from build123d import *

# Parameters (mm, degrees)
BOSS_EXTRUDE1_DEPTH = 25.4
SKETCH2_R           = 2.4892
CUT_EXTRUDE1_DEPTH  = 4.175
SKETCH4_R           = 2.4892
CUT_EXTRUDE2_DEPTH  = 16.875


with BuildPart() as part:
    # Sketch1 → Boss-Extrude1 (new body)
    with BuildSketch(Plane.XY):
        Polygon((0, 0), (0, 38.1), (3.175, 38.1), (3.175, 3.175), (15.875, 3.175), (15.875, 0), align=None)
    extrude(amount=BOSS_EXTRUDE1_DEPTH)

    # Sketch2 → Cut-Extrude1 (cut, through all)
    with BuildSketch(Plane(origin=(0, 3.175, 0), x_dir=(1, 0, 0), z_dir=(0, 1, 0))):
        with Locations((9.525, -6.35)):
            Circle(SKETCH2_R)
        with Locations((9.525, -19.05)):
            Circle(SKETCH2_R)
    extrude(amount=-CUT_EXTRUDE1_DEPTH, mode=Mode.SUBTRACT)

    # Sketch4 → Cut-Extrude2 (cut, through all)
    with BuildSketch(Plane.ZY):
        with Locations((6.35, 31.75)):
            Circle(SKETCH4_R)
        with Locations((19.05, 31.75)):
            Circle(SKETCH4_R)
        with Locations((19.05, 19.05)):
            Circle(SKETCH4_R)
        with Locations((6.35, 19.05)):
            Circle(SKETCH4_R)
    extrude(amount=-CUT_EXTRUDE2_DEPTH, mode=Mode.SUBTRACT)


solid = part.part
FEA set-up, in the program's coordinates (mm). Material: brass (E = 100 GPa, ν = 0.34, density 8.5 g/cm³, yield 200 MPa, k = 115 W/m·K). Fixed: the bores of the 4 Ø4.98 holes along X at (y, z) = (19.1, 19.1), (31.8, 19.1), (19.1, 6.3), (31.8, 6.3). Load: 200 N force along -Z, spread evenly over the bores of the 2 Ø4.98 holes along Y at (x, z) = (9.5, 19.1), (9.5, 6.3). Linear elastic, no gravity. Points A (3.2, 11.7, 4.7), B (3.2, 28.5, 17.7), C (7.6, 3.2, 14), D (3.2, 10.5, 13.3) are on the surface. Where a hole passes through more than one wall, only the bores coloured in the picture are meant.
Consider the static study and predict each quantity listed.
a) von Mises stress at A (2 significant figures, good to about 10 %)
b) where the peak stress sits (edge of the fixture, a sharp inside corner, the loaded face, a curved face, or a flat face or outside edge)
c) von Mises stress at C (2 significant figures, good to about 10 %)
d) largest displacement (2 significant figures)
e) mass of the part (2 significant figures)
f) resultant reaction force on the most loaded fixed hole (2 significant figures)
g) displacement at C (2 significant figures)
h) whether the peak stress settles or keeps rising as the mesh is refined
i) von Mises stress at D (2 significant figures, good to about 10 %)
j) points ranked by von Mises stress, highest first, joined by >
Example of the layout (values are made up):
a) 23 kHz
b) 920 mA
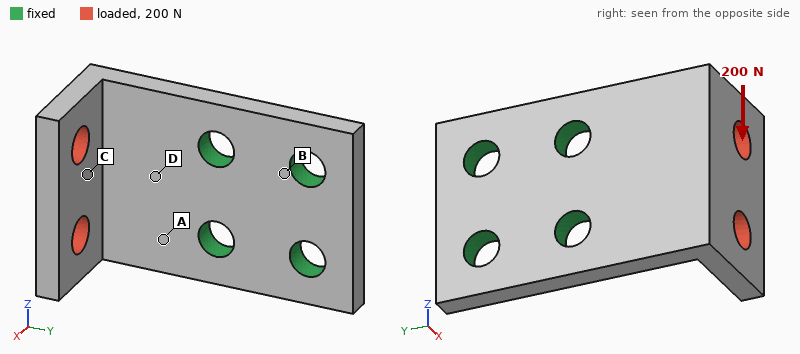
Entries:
a) 21 MPa
b) edge of the fixture
c) 12 MPa
d) 29 µm
e) 32 g
f) 230 N
g) 11 µm
h) keeps rising
i) 27 MPa
j) D > A > C > B
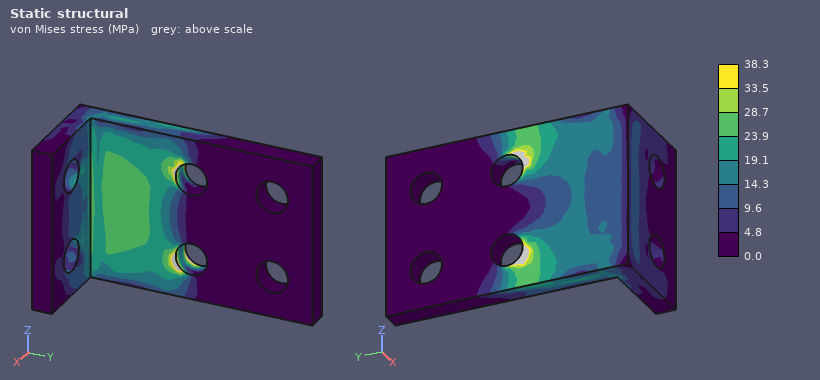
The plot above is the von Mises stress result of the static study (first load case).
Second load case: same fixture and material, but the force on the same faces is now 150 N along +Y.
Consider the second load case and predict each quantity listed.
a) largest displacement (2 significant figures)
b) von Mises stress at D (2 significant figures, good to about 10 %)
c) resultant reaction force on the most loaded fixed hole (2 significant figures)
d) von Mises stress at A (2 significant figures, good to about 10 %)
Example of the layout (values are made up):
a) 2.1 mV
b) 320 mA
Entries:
a) 51 µm
b) 27 MPa
c) 71 N
d) 28 MPa
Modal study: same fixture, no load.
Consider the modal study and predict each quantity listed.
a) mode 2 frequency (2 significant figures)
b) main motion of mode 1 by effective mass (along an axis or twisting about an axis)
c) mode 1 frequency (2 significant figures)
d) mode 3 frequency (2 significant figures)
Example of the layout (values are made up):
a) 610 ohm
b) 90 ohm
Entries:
a) 4700 Hz
b) along X
c) 2700 Hz
d) 7600 Hz
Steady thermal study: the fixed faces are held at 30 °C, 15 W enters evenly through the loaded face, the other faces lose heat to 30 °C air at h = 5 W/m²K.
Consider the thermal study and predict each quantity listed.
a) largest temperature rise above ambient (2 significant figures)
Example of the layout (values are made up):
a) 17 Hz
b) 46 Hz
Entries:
a) 41 K
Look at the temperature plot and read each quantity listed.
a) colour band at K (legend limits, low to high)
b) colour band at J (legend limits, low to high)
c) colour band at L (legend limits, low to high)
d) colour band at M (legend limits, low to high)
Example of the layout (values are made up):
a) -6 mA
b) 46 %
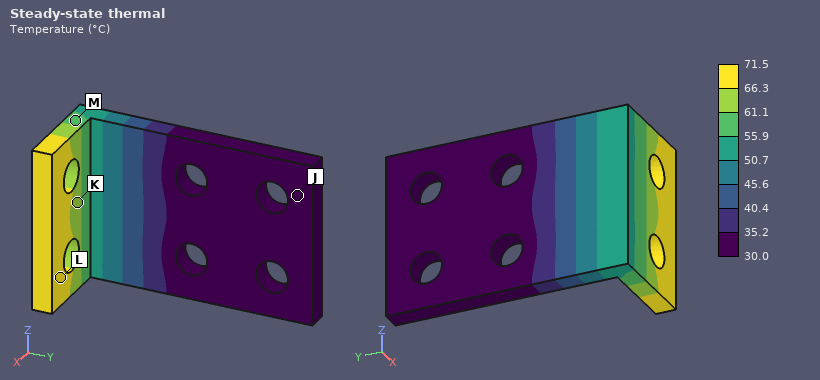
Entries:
a) 61.1 to 66.3 °C
b) 30.0 to 35.2 °C
c) 66.3 to 71.5 °C
d) 55.9 to 61.1 °C
